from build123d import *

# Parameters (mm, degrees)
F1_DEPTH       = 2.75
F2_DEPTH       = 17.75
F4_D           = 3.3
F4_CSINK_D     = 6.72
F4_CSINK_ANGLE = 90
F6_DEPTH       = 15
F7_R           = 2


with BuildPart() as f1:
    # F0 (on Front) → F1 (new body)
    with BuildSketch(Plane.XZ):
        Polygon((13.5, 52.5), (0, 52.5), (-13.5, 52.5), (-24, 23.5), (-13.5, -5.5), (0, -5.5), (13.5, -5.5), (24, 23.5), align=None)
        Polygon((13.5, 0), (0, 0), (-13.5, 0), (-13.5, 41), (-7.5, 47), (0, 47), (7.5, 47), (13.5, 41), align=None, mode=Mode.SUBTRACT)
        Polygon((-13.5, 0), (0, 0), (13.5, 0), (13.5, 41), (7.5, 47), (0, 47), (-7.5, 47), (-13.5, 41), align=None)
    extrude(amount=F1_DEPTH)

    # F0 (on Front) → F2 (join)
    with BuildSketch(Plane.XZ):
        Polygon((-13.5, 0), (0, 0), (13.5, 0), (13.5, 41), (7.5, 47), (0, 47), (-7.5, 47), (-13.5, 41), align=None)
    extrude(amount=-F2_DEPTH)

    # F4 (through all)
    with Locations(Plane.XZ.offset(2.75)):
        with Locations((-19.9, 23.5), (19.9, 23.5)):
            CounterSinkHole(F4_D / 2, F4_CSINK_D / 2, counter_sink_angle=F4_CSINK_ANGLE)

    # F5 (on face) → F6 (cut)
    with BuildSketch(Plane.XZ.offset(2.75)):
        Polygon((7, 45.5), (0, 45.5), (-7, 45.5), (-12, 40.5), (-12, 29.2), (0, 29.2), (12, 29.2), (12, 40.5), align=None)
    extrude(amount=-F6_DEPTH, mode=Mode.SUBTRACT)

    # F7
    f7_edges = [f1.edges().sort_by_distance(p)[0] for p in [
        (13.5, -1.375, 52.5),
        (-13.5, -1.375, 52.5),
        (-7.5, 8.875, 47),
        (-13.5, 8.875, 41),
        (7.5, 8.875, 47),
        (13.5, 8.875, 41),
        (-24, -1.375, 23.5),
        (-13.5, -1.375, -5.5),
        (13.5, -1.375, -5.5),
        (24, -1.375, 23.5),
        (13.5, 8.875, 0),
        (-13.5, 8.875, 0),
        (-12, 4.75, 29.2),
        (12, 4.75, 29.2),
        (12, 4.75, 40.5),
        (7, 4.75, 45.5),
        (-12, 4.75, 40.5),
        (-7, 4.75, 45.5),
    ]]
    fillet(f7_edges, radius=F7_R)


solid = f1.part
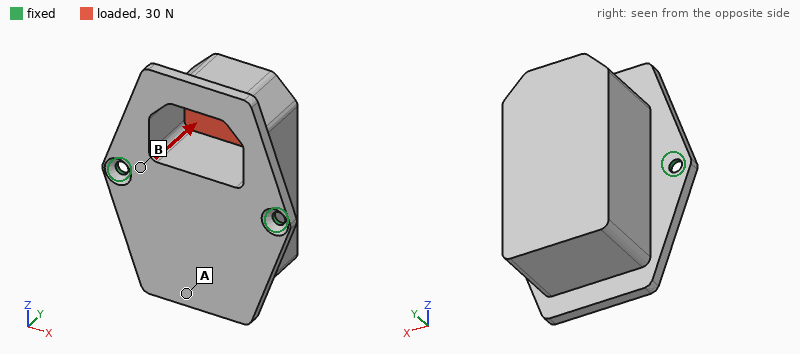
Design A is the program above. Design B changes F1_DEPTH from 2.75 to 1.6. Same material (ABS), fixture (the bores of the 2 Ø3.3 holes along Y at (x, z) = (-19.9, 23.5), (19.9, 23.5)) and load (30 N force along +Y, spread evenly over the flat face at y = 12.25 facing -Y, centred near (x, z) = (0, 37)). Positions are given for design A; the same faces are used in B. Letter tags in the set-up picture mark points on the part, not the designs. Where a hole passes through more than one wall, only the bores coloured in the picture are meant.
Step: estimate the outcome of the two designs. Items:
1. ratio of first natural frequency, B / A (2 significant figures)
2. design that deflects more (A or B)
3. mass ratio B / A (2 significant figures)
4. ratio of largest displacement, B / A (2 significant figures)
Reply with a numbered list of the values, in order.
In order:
1. 0.74
2. B
3. 0.91
4. 2.0
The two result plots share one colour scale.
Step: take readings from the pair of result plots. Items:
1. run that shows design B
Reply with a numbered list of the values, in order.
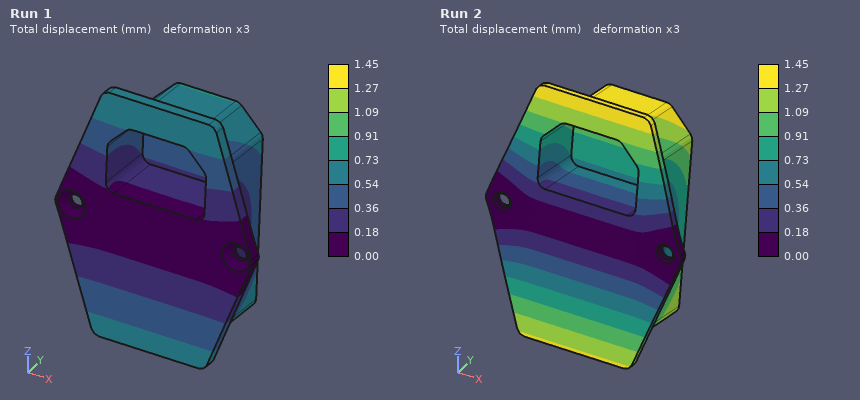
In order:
1. Run 2
